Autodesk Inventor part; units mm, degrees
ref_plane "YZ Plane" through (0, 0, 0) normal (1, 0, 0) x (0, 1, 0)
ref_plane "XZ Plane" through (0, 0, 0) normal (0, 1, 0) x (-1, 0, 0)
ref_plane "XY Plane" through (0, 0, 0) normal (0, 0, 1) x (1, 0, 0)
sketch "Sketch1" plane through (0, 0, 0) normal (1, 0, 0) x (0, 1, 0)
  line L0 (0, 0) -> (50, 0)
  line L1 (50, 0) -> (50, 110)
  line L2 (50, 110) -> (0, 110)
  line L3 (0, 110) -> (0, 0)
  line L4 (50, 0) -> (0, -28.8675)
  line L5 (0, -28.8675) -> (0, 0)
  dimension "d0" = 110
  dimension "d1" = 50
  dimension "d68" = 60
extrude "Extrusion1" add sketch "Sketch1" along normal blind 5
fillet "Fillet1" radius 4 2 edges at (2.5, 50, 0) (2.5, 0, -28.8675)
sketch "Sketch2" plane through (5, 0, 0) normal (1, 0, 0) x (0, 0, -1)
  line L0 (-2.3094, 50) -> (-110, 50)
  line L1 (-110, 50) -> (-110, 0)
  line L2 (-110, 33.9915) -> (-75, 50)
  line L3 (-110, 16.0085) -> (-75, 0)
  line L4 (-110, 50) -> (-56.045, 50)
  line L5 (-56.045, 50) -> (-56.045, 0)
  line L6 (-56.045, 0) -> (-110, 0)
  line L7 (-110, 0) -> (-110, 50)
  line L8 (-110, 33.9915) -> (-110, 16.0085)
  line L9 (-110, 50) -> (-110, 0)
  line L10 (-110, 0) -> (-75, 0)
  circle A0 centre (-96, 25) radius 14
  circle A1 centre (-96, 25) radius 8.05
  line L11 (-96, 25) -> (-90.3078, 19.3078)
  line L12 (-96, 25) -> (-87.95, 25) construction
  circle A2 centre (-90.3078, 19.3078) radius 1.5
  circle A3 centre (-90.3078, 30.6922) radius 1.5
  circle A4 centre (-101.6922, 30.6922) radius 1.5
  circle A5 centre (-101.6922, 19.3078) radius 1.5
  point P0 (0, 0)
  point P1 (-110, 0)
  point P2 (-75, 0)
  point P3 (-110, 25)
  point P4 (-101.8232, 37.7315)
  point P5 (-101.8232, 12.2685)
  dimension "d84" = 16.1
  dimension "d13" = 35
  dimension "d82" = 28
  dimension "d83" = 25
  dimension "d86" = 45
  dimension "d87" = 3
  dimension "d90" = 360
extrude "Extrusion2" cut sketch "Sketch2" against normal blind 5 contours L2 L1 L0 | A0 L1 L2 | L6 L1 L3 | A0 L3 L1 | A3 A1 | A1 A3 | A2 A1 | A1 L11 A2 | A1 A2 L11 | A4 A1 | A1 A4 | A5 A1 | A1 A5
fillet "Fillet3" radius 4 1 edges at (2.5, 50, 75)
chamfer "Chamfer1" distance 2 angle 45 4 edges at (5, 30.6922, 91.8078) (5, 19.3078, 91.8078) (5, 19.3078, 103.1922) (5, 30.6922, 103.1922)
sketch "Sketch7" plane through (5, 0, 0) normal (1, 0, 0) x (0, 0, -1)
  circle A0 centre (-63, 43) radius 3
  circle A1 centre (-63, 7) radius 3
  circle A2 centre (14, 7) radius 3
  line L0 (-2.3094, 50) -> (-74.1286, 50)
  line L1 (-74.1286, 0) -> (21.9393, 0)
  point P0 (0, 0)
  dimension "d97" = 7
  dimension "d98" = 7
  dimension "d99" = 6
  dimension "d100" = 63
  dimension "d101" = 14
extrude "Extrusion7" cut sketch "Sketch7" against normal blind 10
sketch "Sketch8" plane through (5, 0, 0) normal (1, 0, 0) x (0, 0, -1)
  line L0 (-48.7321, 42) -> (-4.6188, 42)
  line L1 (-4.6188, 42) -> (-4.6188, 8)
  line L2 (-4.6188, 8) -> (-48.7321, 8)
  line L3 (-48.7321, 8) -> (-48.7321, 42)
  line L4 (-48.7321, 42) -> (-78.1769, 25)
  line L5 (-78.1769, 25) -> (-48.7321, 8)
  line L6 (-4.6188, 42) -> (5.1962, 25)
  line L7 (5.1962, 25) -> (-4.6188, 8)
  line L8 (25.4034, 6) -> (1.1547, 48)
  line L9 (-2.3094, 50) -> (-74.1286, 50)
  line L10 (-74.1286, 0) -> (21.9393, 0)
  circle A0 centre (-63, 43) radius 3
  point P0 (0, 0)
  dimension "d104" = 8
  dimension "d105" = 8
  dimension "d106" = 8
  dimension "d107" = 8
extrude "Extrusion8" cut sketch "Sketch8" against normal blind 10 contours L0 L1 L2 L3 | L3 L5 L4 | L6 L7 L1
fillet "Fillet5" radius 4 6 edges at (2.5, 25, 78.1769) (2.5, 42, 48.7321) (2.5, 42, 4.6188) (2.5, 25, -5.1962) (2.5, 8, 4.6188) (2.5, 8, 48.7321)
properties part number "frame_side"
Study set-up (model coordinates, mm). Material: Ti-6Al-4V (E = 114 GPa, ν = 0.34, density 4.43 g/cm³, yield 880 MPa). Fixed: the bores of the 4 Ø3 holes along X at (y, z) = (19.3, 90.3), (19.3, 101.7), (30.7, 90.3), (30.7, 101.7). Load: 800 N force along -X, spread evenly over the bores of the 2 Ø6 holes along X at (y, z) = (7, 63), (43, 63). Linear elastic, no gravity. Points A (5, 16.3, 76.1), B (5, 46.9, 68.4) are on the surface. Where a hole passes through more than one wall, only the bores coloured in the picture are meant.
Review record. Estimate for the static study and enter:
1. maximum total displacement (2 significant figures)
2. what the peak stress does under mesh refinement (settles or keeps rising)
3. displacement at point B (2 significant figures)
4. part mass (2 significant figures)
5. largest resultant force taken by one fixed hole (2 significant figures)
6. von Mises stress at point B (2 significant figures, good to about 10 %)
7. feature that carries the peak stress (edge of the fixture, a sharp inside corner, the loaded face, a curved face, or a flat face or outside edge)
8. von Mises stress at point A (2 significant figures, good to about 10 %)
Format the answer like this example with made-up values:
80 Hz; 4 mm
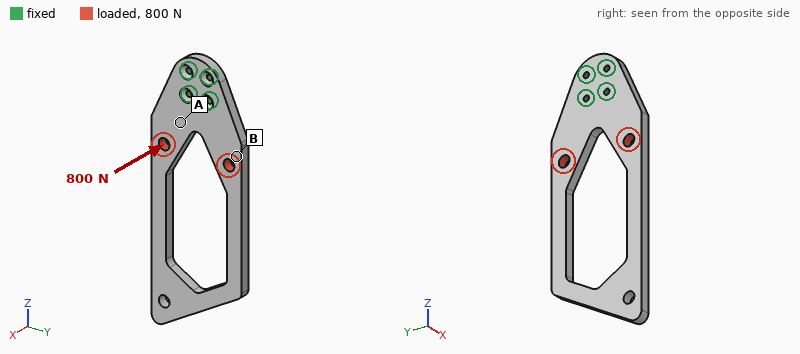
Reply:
0.89 mm; keeps rising; 0.14 mm; 74 g; 1.1 kN; 27 MPa; edge of the fixture; 58 MPa
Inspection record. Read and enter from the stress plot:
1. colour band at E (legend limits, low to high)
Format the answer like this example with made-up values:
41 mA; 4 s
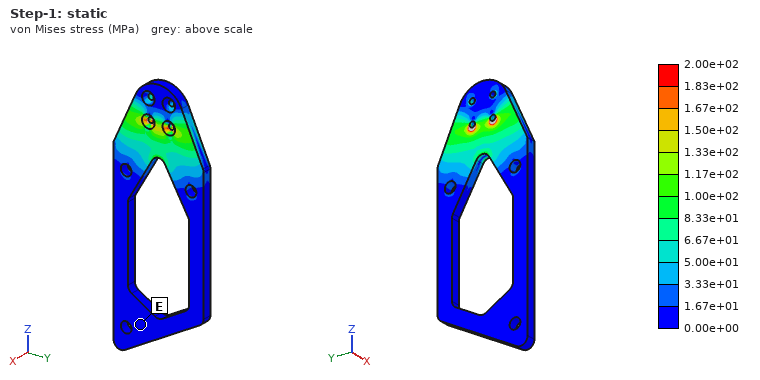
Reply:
0.00e+00 to 1.67e+01 MPa
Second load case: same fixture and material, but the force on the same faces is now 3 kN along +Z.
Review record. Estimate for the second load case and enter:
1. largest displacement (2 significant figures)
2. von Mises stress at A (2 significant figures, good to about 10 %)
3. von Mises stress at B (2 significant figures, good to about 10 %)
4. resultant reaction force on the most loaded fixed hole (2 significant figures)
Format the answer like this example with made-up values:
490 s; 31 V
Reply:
22 µm; 22 MPa; 22 MPa; 970 N
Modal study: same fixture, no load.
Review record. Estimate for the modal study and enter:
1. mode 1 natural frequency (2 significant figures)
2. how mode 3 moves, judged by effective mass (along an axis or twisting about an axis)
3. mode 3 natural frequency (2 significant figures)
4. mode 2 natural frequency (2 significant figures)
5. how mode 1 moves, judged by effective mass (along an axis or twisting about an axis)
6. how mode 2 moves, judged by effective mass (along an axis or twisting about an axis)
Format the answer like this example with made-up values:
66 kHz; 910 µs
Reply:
330 Hz; along Y; 1400 Hz; 1100 Hz; along X; twisting about Z
